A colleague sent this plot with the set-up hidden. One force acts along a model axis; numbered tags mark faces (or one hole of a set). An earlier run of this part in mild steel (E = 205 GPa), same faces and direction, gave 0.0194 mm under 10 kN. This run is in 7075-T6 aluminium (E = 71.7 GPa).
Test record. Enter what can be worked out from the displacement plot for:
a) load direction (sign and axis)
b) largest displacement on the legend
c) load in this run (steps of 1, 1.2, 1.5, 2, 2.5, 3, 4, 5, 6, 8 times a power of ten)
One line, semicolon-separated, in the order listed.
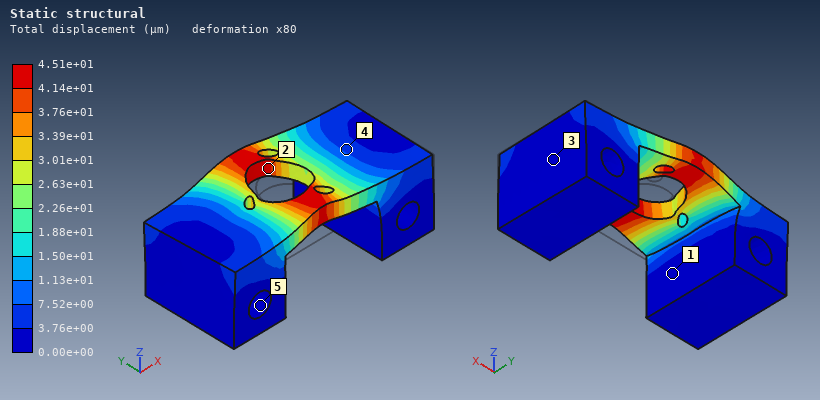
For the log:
+Y; 4.51e+01 µm; 8 kN
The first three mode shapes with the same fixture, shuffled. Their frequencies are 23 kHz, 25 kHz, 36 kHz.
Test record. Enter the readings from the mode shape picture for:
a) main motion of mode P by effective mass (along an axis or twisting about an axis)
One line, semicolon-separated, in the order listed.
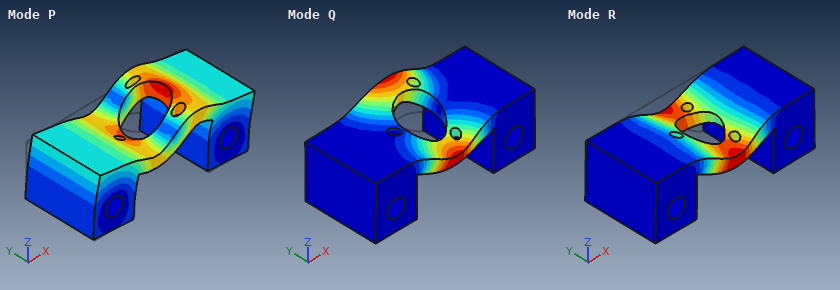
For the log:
along X
